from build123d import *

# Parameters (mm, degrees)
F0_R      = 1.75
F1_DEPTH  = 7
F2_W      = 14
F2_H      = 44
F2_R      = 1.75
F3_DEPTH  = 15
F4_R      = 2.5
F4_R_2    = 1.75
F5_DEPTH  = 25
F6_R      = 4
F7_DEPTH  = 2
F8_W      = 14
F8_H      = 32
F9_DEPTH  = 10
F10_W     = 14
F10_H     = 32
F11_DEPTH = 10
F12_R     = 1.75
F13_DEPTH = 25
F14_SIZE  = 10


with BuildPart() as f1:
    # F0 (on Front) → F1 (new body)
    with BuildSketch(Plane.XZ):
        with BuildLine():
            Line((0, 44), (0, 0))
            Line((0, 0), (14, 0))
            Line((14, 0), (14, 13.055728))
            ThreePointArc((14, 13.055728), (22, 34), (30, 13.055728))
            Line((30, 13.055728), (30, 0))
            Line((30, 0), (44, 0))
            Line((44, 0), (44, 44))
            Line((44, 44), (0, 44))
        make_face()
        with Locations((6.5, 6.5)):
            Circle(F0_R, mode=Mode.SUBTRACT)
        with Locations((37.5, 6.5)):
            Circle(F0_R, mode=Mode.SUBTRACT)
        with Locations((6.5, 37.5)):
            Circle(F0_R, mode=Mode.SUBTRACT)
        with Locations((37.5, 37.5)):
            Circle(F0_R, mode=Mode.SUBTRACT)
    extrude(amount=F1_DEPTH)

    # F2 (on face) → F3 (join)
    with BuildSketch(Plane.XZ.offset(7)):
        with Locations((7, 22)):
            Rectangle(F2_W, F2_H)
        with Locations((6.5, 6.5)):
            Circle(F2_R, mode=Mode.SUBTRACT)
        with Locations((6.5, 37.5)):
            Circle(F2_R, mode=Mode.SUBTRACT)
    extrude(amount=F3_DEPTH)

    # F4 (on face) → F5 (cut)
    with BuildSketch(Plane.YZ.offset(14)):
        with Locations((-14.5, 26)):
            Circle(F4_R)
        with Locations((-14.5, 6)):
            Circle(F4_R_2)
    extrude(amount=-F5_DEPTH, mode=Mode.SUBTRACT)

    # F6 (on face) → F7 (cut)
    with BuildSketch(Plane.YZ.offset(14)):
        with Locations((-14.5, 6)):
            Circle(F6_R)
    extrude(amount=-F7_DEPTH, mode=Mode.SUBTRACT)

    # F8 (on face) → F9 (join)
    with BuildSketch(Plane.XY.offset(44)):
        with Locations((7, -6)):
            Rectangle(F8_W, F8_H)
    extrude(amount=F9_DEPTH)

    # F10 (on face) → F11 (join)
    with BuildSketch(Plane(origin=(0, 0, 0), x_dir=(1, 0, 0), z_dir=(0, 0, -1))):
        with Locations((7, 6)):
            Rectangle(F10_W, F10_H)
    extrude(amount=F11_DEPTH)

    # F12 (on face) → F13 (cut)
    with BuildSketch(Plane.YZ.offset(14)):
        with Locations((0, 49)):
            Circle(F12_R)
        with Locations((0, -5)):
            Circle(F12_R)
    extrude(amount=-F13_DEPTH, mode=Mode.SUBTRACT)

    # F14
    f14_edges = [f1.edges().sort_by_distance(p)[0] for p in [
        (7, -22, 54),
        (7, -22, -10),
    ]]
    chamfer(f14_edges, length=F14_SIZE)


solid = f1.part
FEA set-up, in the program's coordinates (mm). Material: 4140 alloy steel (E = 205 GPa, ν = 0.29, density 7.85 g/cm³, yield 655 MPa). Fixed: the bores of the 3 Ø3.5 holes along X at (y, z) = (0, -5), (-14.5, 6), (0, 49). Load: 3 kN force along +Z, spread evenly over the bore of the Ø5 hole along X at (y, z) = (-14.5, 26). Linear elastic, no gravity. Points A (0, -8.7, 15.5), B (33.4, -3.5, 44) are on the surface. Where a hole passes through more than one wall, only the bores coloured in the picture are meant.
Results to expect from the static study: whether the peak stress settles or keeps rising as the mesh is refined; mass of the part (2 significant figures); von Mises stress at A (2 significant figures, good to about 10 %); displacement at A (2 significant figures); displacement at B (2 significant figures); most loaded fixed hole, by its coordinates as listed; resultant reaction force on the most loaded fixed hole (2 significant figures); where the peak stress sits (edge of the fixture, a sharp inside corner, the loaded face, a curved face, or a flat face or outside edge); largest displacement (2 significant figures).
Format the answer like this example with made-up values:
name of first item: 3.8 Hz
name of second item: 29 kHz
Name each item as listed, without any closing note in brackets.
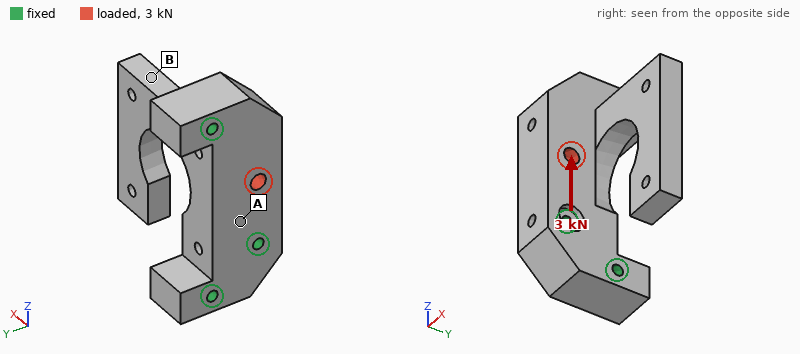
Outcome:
whether the peak stress settles or keeps rising as the mesh is refined: keeps rising
mass of the part: 190 g
von Mises stress at A: 7.7 MPa
displacement at A: 0.61 µm
displacement at B: 0.59 µm
most loaded fixed hole, by its coordinates as listed: (-14.5, 6)
resultant reaction force on the most loaded fixed hole: 1.7 kN
where the peak stress sits: edge of the fixture
largest displacement: 1.8 µm
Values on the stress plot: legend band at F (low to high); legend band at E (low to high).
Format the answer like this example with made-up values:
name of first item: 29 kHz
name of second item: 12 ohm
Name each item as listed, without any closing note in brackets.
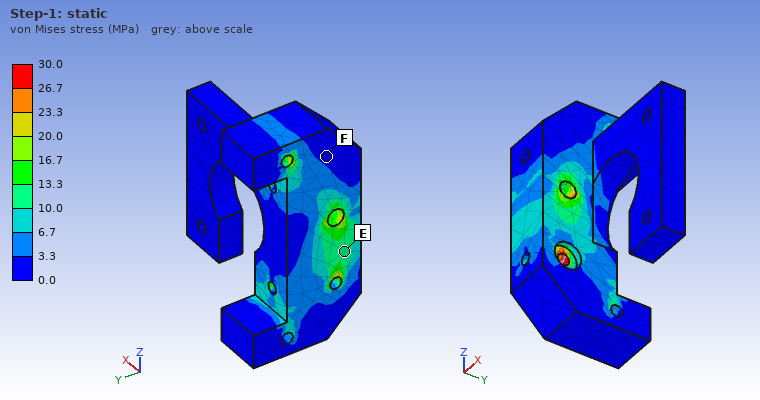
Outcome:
legend band at F: 0.0 to 3.3 MPa
legend band at E: 10.0 to 13.3 MPa
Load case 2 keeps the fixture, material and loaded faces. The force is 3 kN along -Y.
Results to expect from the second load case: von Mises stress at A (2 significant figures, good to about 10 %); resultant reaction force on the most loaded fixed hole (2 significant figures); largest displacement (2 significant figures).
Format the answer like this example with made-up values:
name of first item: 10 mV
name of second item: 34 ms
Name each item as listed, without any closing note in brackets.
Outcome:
von Mises stress at A: 15 MPa
resultant reaction force on the most loaded fixed hole: 1.7 kN
largest displacement: 6.7 µm
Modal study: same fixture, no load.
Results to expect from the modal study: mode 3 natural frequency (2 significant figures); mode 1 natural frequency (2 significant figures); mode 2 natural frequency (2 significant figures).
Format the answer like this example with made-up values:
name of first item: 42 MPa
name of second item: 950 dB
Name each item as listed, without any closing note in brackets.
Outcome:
mode 3 natural frequency: 4500 Hz
mode 1 natural frequency: 1700 Hz
mode 2 natural frequency: 2500 Hz
